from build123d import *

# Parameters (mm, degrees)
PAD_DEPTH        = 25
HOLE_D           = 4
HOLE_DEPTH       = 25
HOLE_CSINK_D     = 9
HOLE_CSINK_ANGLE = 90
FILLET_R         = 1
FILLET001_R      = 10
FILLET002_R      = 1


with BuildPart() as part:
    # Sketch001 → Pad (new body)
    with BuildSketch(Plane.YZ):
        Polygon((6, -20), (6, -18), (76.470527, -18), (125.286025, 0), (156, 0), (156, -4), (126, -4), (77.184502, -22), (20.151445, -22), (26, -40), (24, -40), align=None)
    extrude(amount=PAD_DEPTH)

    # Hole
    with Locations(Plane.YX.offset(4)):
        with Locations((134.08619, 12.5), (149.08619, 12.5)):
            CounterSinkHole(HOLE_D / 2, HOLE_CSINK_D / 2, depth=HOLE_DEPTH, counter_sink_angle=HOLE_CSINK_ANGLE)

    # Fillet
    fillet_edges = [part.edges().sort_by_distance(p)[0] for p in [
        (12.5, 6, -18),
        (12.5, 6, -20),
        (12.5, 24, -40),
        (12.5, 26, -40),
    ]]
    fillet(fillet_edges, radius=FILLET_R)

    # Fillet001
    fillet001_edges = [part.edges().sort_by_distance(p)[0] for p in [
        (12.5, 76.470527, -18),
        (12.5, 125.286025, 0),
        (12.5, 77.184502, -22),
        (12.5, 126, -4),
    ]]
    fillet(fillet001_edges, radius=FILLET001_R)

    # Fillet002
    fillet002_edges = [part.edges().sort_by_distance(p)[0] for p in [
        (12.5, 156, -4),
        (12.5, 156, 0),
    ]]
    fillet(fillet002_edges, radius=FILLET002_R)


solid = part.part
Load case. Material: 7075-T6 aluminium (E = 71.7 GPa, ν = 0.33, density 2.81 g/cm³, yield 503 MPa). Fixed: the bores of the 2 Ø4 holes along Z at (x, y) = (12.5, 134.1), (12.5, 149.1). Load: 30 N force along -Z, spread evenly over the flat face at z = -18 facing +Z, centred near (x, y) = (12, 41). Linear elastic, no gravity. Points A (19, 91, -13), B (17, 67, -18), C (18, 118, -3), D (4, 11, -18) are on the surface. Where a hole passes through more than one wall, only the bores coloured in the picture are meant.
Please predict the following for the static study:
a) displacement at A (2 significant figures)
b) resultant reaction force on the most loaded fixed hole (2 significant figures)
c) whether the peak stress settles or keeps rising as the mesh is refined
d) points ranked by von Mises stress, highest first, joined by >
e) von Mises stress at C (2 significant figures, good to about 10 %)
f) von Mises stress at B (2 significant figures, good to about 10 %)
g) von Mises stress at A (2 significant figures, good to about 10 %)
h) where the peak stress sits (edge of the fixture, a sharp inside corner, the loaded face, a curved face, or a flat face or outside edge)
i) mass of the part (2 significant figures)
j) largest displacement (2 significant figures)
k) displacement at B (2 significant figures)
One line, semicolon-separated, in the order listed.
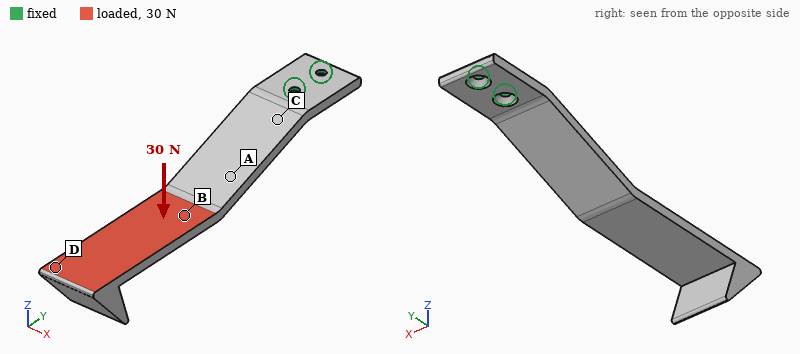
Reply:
0.30 mm; 260 N; keeps rising; C > A > B > D; 34 MPa; 12 MPa; 23 MPa; edge of the fixture; 51 g; 1.5 mm; 0.61 mm
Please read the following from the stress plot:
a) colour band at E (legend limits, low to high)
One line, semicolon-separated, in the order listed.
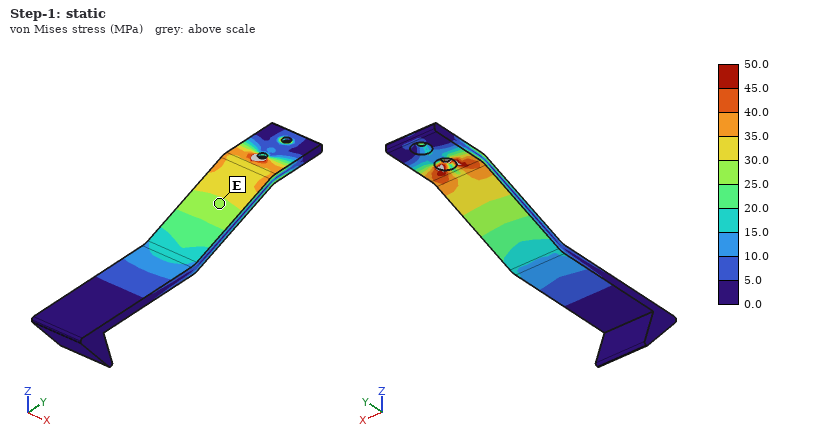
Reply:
25.0 to 30.0 MPa
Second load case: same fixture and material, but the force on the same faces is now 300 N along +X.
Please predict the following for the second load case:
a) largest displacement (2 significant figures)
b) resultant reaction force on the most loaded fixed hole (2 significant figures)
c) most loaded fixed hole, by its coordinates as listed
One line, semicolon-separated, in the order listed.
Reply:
1.0 mm; 1.8 kN; (12.5, 134.1)
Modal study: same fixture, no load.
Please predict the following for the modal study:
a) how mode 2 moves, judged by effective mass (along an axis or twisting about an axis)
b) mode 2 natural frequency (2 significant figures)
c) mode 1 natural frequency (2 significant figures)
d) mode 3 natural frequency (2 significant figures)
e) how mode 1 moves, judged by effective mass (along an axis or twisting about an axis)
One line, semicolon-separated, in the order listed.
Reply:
along X; 570 Hz; 140 Hz; 980 Hz; along Z
